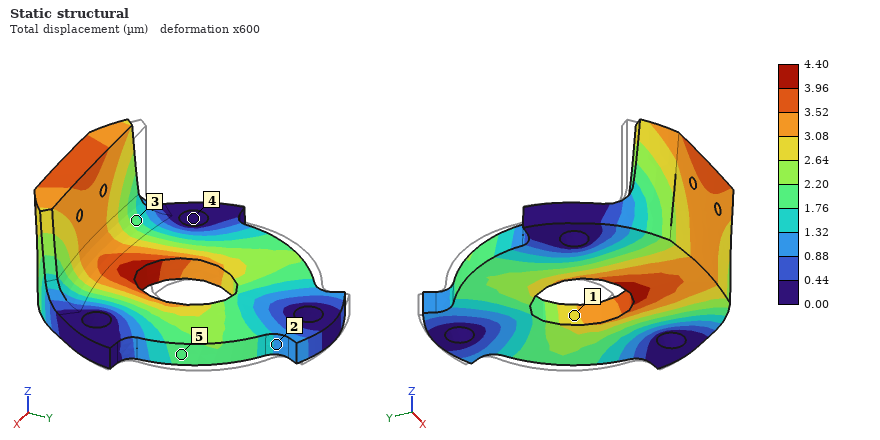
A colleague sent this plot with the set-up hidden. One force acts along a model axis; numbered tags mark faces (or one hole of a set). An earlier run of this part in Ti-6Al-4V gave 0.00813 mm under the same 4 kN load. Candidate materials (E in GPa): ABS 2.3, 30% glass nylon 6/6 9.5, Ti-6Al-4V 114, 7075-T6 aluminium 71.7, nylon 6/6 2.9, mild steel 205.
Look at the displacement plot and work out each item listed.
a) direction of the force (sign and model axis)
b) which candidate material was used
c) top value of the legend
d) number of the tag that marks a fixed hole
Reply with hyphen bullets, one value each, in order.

- -Y
- mild steel
- 4.40 µm
- 4
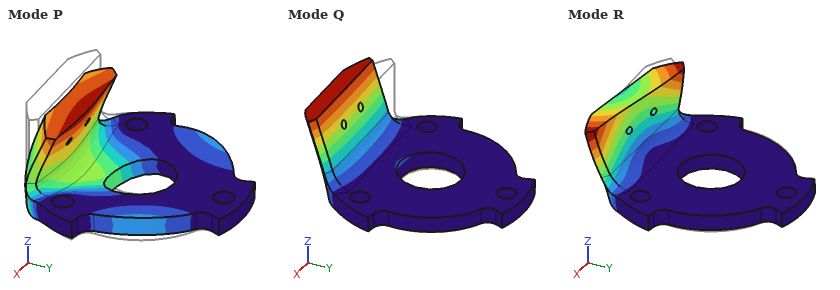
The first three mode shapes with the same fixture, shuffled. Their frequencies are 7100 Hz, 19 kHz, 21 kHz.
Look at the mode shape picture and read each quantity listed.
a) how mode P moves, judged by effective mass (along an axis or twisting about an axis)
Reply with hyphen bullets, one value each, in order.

- along Z
